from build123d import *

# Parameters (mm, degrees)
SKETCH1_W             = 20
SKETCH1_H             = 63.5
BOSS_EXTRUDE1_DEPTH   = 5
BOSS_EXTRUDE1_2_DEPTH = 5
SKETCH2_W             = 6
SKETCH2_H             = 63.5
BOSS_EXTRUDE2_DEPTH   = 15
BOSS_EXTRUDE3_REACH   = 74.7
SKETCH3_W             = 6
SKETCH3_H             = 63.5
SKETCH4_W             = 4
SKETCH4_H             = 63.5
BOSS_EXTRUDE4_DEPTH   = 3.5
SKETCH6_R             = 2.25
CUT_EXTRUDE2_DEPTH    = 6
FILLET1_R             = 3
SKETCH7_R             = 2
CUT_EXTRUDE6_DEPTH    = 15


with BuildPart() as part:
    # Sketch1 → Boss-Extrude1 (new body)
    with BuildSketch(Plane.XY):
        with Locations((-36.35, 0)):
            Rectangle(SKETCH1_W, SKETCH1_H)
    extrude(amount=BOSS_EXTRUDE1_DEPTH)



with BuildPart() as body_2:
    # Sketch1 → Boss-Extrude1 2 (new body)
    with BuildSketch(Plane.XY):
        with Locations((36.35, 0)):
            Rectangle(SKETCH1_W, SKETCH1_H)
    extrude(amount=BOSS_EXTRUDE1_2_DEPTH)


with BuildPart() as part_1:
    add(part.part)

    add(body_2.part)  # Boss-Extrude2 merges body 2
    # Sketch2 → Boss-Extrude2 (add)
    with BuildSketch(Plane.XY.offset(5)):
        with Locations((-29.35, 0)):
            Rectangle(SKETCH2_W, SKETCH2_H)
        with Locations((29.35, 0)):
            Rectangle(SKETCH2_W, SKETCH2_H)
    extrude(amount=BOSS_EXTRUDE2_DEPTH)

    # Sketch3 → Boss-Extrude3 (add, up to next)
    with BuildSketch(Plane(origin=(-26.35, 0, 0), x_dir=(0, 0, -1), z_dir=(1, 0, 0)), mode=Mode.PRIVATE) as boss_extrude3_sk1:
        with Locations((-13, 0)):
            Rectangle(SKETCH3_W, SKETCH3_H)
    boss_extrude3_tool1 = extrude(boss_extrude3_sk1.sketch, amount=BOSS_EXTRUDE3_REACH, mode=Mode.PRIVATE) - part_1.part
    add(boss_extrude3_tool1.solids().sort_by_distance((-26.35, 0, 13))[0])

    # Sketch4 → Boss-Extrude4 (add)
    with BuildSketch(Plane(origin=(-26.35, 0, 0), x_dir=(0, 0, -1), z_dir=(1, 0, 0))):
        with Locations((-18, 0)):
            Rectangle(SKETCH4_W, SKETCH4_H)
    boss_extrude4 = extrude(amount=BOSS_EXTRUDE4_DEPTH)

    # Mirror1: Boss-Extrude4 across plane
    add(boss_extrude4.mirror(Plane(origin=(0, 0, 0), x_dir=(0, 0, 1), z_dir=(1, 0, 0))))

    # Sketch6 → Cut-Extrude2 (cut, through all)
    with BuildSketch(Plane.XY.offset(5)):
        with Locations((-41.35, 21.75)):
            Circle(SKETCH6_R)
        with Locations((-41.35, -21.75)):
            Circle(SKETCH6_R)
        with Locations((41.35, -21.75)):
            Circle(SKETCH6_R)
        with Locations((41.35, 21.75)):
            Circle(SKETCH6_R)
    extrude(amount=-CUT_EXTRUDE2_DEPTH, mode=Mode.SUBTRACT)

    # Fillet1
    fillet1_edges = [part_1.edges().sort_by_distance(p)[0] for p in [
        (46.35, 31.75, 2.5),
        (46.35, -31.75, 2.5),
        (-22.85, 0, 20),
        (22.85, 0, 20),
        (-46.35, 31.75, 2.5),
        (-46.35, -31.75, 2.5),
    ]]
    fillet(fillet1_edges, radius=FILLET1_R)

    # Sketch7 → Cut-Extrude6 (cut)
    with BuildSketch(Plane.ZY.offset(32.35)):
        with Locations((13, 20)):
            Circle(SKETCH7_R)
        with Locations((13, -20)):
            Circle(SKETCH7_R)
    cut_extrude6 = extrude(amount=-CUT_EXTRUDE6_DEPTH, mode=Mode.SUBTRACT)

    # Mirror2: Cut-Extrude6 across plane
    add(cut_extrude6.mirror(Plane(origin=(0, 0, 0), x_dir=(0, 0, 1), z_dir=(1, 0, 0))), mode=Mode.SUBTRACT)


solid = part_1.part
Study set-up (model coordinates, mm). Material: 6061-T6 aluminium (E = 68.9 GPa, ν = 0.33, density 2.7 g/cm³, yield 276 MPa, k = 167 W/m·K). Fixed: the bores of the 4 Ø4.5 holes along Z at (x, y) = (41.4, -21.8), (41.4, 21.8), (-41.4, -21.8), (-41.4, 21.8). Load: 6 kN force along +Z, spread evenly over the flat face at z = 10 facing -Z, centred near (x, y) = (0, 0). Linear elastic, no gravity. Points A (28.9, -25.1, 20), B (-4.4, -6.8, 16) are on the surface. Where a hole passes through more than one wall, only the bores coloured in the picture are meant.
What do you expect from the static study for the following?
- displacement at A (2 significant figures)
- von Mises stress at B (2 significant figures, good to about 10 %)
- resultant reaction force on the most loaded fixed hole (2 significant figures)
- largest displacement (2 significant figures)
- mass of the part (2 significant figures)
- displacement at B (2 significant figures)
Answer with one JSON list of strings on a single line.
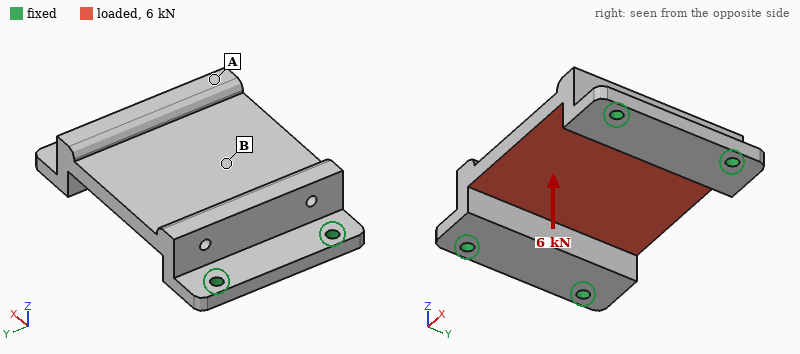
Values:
["30 µm", "52 MPa", "2.8 kN", "88 µm", "120 g", "80 µm"]
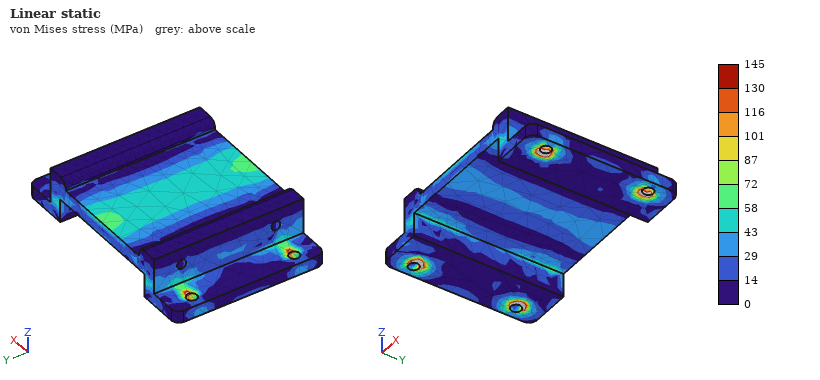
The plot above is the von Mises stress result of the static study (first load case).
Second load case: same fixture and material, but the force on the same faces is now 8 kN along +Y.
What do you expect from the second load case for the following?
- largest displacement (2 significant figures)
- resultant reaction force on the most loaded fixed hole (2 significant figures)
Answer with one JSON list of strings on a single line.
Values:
["28 µm", "2.4 kN"]
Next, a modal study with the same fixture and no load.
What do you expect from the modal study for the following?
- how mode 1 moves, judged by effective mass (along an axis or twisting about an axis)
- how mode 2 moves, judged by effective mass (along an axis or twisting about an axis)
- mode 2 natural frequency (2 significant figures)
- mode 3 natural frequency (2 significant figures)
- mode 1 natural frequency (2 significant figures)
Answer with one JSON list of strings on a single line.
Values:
["along Z", "along X", "6600 Hz", "7000 Hz", "6000 Hz"]
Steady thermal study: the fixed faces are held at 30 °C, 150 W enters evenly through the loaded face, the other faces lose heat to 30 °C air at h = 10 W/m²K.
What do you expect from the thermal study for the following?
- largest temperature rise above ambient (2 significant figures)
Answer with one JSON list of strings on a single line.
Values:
["50 K"]
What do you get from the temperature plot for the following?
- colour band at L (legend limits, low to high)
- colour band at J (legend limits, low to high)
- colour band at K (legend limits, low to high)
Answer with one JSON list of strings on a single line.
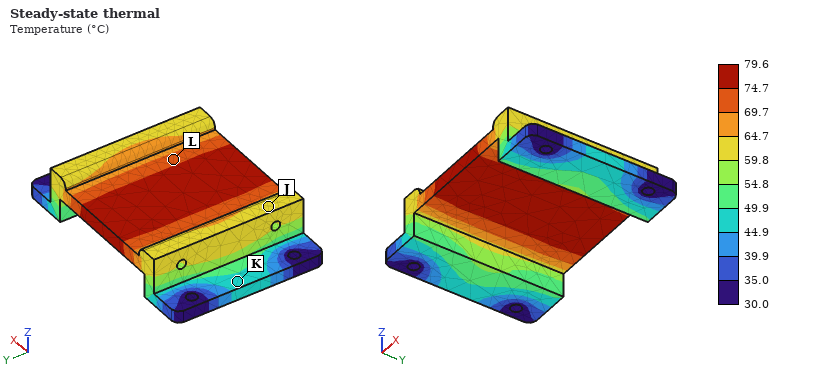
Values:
["69.7 to 74.7 °C", "59.8 to 64.7 °C", "44.9 to 49.9 °C"]
